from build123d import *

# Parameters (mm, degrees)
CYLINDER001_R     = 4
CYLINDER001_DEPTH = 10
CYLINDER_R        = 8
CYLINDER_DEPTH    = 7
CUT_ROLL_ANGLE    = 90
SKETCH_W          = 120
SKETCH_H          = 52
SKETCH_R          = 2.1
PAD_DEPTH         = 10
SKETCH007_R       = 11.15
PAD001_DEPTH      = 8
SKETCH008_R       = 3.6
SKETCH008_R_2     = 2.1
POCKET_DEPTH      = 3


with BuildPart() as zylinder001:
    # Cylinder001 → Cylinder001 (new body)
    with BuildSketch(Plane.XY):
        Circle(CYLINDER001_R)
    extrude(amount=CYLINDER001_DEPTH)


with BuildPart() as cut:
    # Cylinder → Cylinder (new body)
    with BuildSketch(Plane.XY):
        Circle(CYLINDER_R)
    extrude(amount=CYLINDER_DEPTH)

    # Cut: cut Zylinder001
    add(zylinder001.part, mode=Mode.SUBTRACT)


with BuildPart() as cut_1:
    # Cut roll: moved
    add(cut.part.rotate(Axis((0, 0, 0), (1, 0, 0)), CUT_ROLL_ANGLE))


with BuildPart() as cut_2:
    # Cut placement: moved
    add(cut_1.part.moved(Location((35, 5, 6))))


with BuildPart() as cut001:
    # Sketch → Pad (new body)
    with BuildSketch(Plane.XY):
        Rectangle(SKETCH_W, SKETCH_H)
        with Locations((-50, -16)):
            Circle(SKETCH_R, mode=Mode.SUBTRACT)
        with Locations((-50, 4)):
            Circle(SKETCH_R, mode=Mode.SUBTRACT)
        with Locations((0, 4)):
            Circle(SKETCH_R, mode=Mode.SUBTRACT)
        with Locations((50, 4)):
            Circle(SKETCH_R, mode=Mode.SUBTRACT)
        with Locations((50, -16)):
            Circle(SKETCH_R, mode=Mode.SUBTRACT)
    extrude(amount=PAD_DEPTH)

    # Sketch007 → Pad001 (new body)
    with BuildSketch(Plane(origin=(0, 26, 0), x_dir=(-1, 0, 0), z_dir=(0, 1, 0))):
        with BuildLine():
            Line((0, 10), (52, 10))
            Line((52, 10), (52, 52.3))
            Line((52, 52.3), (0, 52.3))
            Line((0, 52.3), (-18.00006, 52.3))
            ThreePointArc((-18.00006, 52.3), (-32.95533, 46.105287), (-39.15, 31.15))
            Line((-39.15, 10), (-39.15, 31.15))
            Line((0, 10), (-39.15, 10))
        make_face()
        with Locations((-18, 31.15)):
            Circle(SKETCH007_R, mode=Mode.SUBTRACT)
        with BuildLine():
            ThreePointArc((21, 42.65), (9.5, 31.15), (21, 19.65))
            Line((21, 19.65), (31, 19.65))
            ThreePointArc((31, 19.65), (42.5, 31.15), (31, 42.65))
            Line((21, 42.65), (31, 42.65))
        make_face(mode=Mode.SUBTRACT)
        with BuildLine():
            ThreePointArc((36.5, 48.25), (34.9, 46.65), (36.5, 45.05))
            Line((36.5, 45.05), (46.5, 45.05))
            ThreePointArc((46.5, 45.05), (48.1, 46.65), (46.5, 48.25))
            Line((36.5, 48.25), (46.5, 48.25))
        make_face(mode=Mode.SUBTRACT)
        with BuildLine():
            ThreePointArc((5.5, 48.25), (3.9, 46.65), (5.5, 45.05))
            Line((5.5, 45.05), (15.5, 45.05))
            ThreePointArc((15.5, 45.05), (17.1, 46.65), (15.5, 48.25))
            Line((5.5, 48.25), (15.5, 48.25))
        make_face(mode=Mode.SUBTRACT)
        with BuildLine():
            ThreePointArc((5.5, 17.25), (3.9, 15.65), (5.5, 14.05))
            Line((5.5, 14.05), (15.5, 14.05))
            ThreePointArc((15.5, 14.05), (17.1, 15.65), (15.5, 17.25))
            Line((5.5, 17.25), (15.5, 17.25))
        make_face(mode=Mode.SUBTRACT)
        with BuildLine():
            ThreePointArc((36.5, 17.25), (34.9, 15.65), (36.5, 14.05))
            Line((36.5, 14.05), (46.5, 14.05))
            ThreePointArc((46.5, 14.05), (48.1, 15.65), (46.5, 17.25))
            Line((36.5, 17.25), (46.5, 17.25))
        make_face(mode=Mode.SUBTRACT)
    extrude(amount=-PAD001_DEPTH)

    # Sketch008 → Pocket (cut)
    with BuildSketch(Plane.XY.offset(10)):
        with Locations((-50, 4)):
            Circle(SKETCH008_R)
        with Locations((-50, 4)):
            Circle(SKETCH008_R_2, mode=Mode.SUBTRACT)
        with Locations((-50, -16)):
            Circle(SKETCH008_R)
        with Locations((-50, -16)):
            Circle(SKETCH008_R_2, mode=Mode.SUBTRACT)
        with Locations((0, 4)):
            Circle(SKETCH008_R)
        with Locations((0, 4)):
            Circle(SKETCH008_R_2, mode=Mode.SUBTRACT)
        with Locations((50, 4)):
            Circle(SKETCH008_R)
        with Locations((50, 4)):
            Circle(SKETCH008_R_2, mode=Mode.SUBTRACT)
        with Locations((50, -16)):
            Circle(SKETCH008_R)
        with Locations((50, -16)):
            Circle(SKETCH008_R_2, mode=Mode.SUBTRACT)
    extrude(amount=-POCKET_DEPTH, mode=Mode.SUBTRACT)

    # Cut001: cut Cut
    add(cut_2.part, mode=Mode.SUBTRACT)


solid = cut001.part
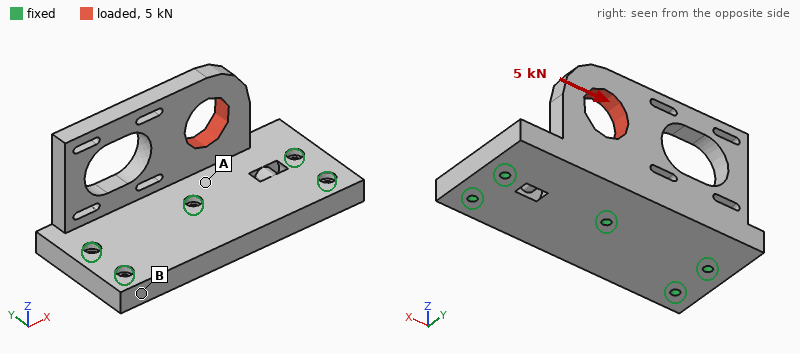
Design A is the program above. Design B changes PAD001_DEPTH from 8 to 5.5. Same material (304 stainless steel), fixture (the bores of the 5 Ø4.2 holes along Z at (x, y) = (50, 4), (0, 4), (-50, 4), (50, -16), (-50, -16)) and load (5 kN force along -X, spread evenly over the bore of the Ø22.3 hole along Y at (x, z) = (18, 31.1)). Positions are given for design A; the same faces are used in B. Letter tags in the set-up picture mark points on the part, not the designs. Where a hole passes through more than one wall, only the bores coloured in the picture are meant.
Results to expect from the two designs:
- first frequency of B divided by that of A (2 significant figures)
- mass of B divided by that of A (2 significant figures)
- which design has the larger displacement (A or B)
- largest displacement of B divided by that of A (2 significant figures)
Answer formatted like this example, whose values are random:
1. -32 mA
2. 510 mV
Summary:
1. 0.82
2. 0.92
3. B
4. 1.3
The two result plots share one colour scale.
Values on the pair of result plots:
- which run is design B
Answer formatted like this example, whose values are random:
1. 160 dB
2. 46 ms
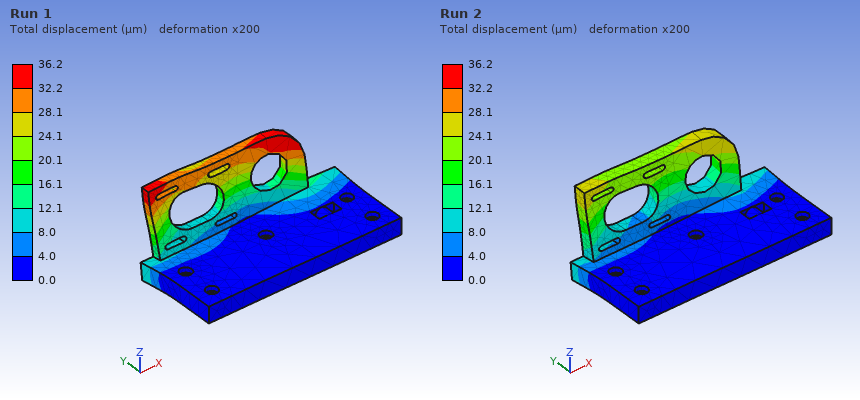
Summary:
1. Run 1
